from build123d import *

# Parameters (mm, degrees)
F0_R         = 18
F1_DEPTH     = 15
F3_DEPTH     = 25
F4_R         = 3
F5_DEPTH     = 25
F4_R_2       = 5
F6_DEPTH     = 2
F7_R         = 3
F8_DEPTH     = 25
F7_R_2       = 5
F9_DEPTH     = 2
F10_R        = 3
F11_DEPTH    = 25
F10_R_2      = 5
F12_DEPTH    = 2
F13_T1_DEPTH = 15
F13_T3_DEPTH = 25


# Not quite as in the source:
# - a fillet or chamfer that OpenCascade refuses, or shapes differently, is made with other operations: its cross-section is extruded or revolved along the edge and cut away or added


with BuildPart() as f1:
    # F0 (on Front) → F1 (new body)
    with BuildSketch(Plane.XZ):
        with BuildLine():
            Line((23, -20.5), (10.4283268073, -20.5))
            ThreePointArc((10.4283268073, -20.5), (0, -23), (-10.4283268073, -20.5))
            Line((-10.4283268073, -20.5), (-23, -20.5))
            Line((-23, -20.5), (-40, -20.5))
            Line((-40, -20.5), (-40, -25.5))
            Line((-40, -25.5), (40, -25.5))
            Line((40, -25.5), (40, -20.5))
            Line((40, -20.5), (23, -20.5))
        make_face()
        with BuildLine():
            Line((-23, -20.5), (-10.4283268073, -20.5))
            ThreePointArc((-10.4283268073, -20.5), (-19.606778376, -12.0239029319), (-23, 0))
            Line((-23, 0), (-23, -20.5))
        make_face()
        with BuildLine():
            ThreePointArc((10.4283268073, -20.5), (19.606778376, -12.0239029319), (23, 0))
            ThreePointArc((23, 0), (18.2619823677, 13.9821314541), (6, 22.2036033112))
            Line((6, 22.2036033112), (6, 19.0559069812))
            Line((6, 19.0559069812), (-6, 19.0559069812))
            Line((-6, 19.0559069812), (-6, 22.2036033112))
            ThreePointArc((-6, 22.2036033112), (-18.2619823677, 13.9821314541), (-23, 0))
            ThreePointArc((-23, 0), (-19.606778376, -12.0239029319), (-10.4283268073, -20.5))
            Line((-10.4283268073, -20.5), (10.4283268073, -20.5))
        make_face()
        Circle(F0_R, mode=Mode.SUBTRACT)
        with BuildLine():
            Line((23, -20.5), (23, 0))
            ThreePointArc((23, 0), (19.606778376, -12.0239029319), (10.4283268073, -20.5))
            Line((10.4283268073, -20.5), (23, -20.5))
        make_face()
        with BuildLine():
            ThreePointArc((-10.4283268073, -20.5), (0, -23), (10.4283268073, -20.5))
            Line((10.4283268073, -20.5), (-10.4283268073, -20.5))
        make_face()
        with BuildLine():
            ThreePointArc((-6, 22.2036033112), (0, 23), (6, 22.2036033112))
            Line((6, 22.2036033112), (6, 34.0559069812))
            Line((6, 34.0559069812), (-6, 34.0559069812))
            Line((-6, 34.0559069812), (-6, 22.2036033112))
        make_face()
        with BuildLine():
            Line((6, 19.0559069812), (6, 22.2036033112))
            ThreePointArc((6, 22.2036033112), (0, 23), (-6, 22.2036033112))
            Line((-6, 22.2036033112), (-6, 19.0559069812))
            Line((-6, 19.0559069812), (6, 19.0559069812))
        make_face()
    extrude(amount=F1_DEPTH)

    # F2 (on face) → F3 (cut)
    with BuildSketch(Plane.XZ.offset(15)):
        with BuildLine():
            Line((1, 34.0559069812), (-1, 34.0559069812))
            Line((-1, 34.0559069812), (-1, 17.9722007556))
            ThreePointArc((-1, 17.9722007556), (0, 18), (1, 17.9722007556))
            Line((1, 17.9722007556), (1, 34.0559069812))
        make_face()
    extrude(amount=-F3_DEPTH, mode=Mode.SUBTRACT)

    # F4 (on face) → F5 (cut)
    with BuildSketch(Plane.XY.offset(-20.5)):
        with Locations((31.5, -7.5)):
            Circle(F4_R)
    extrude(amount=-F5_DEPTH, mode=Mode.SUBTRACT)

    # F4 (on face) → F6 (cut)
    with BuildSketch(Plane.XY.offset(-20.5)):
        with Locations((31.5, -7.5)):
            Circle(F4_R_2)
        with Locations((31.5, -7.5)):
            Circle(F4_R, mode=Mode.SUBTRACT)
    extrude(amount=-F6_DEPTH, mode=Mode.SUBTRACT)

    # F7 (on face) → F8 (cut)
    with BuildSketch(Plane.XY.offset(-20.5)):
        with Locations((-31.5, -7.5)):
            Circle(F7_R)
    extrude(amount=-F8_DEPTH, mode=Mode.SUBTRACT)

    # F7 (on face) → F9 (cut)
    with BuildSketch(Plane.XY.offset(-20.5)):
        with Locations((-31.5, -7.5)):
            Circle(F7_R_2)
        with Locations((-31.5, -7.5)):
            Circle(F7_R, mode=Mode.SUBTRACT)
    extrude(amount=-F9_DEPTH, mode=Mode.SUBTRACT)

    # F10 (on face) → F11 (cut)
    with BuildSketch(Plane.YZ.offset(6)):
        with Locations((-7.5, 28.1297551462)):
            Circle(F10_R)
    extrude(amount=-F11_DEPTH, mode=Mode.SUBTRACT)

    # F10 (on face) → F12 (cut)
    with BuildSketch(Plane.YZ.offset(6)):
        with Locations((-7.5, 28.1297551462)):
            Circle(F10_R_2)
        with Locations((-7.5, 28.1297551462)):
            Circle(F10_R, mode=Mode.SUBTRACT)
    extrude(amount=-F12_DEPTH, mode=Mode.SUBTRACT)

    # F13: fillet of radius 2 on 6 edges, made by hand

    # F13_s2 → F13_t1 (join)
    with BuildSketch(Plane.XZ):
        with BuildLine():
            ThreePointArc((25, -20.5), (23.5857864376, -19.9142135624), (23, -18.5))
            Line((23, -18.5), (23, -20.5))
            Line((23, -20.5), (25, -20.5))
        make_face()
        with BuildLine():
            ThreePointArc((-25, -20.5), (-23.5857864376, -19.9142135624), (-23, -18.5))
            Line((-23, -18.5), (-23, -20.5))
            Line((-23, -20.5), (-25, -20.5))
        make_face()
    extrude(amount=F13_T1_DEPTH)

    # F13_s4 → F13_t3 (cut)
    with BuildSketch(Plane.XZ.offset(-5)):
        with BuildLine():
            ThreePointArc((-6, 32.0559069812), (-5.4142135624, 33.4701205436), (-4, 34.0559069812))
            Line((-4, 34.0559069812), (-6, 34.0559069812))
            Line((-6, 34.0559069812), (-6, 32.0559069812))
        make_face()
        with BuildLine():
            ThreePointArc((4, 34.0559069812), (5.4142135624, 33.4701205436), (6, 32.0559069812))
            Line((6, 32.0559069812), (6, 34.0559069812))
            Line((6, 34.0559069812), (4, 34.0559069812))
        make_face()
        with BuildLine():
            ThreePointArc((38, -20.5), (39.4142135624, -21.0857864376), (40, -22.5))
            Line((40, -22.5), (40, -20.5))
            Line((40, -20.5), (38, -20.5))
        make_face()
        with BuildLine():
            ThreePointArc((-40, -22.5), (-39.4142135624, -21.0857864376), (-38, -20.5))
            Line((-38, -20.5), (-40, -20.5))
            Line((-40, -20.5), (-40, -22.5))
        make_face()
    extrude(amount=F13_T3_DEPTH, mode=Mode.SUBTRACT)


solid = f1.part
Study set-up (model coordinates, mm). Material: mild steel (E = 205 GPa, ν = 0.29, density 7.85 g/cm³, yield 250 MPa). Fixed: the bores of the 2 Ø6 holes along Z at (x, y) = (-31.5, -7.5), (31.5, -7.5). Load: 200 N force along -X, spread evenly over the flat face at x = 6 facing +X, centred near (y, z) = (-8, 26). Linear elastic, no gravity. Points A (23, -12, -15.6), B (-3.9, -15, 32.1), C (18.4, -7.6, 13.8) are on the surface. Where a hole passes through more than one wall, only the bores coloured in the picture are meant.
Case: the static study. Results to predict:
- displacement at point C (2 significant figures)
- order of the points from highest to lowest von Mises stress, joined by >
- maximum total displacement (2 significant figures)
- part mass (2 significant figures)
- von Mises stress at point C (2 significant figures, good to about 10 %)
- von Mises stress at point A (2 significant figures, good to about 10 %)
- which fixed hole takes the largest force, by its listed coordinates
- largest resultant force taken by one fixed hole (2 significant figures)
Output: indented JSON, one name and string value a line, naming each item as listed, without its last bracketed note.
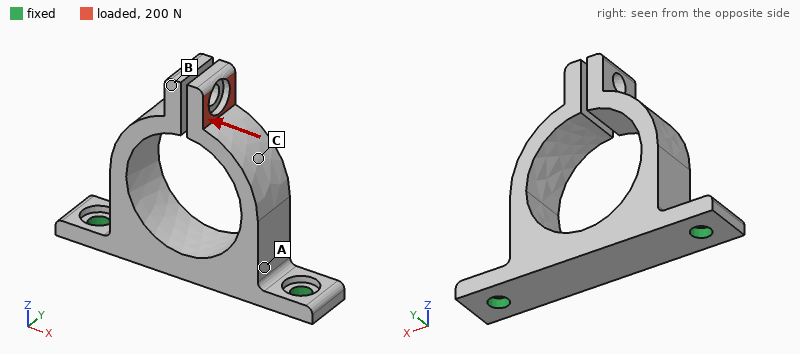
{
  "displacement at point C": "0.059 mm",
  "order of the points from highest to lowest von Mises stress, joined by >": "C > A > B",
  "maximum total displacement": "0.17 mm",
  "part mass": "140 g",
  "von Mises stress at point C": "43 MPa",
  "von Mises stress at point A": "29 MPa",
  "which fixed hole takes the largest force, by its listed coordinates": "(-31.5, -7.5)",
  "largest resultant force taken by one fixed hole": "470 N"
}
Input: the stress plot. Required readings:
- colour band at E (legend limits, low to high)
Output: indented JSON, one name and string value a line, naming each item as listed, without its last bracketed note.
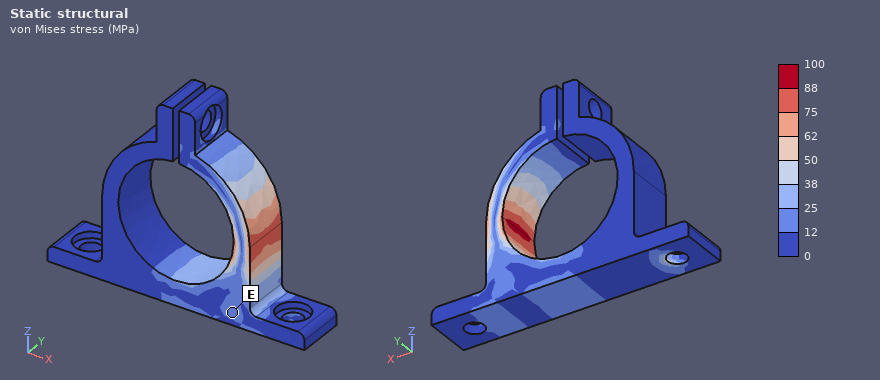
{
  "colour band at E": "12 to 25 MPa"
}
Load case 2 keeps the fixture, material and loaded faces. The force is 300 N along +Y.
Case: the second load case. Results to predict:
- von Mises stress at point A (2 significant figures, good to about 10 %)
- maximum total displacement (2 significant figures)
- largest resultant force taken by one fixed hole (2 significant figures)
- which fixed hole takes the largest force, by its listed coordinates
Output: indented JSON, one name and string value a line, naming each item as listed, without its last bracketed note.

{
  "von Mises stress at point A": "39 MPa",
  "maximum total displacement": "0.20 mm",
  "largest resultant force taken by one fixed hole": "190 N",
  "which fixed hole takes the largest force, by its listed coordinates": "(31.5, -7.5)"
}
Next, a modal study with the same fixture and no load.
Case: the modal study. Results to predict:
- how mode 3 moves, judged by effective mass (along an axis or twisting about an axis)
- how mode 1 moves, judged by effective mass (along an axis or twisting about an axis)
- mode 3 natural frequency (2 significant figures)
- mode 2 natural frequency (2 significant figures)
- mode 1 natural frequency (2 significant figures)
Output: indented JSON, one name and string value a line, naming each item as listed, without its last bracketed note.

{
  "how mode 3 moves, judged by effective mass": "along X",
  "how mode 1 moves, judged by effective mass": "along Y",
  "mode 3 natural frequency": "1800 Hz",
  "mode 2 natural frequency": "1600 Hz",
  "mode 1 natural frequency": "1400 Hz"
}
